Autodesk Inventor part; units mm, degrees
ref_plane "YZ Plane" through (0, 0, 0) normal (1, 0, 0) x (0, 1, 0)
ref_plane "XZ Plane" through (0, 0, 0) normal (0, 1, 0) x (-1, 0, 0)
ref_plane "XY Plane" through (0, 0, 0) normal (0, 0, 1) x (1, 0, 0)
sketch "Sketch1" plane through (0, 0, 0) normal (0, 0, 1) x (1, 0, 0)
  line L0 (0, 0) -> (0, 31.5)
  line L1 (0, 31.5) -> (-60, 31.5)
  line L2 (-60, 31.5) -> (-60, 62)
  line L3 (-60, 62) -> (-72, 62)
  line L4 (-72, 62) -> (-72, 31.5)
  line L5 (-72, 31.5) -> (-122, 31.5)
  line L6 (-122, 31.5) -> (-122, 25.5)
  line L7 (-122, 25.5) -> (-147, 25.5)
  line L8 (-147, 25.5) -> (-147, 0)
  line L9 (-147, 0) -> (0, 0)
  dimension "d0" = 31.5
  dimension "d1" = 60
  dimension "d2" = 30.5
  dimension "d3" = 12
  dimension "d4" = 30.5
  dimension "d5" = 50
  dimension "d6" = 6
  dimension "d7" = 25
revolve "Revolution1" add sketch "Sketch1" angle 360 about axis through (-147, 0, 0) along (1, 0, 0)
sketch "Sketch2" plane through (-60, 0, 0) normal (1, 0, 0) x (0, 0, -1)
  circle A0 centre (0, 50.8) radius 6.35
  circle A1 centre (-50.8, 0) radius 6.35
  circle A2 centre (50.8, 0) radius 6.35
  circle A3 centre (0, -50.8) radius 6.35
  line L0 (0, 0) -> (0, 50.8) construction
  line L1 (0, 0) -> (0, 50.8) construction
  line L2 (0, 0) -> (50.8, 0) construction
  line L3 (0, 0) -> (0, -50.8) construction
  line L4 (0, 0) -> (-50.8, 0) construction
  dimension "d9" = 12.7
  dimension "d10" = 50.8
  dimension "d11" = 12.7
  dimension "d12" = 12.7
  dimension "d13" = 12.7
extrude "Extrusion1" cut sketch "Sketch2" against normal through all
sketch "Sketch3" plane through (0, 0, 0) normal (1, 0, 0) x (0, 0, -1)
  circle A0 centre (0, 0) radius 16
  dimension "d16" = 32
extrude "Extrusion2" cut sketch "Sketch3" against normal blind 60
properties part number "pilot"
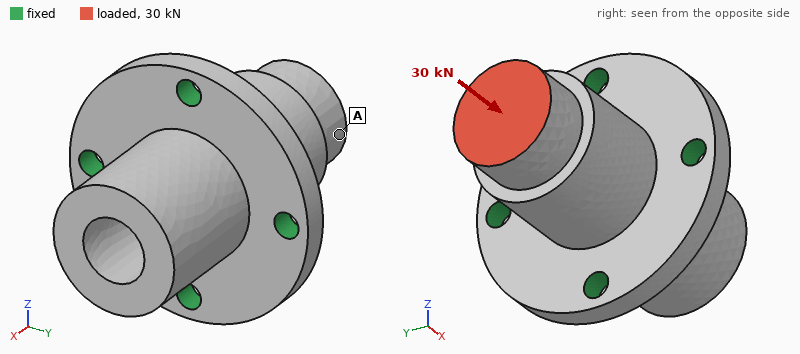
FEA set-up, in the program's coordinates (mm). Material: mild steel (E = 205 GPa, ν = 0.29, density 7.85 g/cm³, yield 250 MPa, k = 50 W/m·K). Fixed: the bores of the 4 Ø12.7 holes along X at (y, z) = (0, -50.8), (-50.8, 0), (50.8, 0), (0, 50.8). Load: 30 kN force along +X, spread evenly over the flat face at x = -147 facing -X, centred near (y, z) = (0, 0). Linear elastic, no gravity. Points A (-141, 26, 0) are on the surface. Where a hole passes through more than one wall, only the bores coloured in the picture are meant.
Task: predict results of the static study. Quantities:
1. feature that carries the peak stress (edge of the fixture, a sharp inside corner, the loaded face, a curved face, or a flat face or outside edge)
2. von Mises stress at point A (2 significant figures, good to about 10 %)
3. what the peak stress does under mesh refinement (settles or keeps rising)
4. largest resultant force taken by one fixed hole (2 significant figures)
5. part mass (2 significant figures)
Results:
edge of the fixture
15 MPa
keeps rising
7.6 kN
3.8 kg
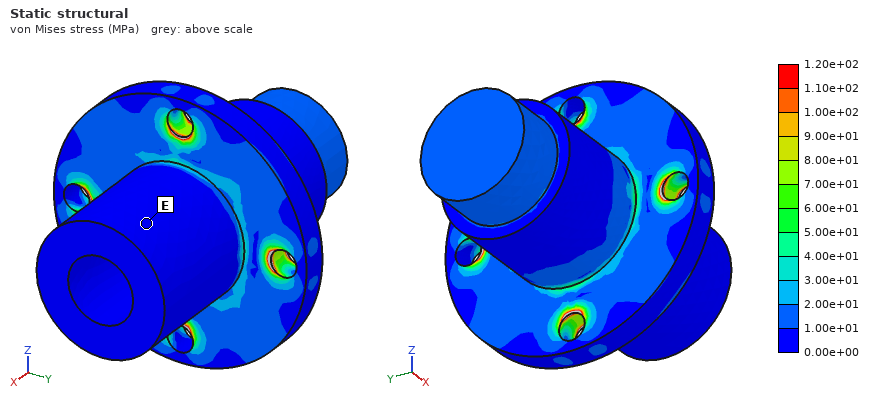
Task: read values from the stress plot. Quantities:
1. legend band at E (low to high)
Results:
0.00e+00 to 1.00e+01 MPa
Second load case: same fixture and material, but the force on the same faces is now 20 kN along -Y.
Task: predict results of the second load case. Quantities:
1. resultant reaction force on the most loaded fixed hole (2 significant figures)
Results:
19 kN
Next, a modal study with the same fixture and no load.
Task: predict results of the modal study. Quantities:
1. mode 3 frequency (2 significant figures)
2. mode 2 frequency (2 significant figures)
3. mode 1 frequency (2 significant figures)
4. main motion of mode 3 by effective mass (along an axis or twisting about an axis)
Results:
4900 Hz
3200 Hz
3100 Hz
along X
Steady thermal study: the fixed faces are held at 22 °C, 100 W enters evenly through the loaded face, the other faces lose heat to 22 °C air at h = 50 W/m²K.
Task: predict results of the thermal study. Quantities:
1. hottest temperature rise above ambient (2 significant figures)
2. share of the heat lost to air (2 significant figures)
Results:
66 K
42 %
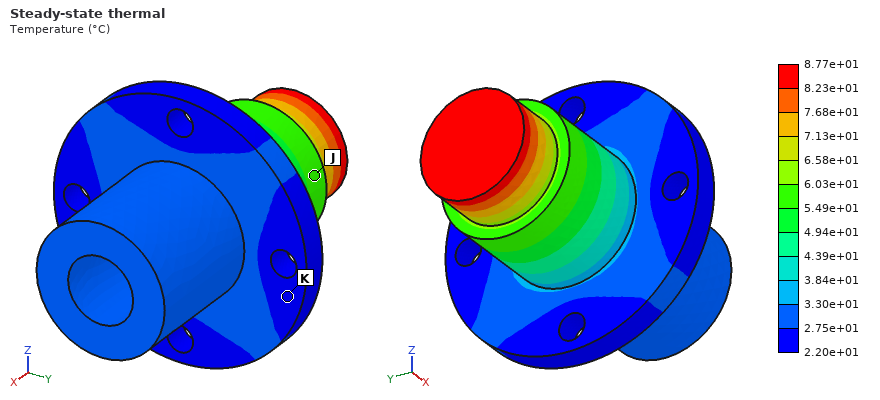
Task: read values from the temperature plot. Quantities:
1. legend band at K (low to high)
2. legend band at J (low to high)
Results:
2.20e+01 to 2.75e+01 °C
5.49e+01 to 6.03e+01 °C
